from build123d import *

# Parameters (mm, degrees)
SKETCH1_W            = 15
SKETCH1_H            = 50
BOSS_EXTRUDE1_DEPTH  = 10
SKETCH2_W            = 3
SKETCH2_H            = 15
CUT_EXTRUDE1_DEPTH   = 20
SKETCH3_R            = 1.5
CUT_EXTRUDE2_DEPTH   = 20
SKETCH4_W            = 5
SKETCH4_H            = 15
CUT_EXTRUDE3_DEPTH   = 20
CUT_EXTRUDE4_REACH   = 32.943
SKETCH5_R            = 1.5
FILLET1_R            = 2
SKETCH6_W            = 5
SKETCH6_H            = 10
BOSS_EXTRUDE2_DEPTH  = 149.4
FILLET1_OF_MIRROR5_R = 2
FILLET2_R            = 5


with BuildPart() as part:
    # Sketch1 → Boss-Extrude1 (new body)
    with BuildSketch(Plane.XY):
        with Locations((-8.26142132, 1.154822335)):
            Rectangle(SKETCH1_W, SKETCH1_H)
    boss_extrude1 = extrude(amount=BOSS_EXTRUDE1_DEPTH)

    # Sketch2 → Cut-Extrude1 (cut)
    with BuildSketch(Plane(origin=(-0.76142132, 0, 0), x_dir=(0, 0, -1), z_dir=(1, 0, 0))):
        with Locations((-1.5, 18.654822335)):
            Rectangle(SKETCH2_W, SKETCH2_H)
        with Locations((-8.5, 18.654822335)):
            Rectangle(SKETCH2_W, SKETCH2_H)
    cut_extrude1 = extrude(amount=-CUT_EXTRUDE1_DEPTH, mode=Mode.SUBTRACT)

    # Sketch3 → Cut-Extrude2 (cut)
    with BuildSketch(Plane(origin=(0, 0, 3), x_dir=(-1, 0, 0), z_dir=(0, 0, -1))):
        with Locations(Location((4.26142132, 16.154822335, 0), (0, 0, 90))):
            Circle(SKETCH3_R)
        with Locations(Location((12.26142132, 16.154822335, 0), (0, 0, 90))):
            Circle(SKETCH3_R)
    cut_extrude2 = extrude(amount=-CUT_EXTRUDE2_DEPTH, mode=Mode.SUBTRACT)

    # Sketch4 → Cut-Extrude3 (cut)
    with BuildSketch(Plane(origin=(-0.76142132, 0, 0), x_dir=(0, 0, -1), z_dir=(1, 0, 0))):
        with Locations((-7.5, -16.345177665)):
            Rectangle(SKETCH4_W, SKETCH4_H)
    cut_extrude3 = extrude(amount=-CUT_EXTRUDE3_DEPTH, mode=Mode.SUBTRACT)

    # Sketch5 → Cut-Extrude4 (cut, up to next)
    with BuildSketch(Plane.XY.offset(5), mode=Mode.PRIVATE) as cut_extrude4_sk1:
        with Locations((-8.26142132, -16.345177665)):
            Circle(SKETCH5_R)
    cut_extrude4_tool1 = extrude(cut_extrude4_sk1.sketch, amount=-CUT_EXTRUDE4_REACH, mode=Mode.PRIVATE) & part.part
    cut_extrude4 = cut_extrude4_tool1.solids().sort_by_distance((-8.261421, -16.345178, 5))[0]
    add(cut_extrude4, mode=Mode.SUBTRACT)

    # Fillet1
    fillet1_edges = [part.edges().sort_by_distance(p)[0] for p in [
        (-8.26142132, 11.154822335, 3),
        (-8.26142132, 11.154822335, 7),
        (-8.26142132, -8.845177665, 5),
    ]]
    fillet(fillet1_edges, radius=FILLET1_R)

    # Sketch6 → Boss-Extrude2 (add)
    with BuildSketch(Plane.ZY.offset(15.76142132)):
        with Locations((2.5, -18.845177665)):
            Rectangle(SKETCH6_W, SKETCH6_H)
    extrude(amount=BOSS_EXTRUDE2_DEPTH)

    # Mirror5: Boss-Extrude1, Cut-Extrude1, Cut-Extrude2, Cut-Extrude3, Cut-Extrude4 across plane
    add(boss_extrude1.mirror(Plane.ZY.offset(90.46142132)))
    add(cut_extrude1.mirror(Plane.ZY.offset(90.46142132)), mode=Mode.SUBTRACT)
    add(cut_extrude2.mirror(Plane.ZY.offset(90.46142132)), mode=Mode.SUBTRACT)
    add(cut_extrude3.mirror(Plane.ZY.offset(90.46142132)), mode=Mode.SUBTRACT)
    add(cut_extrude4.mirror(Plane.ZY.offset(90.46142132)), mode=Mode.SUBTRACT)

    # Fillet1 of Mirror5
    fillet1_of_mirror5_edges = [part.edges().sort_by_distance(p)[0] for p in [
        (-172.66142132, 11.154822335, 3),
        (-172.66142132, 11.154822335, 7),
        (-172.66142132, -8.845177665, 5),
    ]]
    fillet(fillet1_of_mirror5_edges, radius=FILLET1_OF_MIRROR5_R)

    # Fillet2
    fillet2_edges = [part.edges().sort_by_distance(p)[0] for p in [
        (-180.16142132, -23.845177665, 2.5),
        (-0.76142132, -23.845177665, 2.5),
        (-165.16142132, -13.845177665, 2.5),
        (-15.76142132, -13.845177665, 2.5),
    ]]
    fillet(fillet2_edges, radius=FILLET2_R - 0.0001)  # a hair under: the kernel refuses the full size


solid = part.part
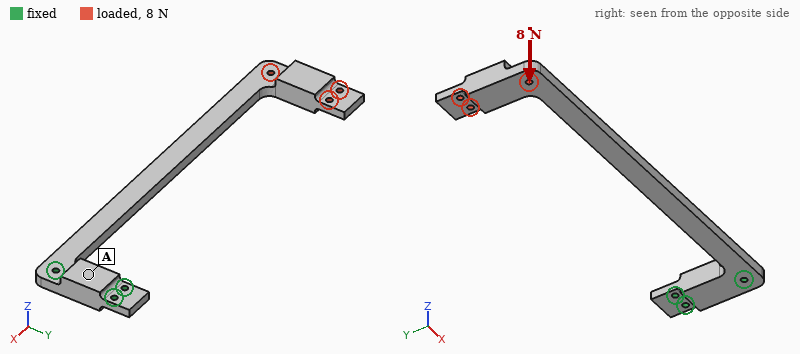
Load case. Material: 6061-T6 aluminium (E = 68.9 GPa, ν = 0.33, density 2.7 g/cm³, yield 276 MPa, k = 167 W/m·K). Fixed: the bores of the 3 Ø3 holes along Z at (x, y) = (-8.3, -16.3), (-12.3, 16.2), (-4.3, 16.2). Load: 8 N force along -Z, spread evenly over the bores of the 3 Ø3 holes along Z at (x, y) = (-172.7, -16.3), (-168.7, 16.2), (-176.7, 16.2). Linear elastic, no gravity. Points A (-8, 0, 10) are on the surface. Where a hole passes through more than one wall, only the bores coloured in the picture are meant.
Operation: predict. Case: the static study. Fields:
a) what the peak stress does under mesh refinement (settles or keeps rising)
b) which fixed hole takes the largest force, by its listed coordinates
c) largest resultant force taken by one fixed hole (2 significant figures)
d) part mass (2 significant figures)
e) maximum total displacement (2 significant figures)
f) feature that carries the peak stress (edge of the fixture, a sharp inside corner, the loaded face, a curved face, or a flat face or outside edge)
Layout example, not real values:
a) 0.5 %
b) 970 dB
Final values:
a) keeps rising
b) (-4.3, 16.2)
c) 30 N
d) 47 g
e) 1.9 mm
f) edge of the fixture
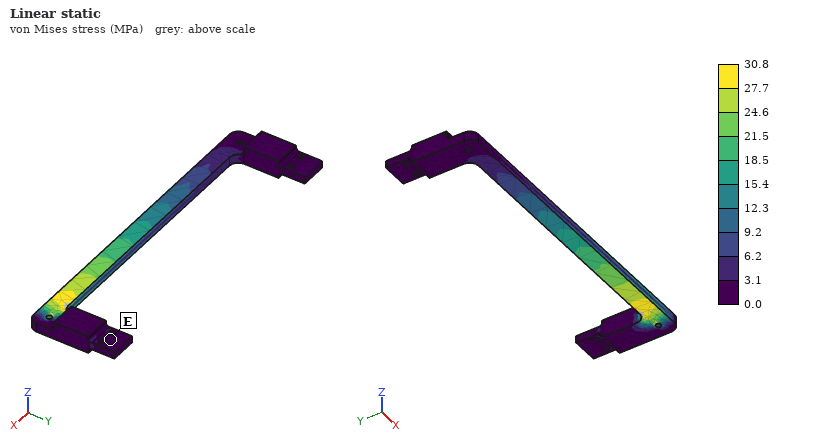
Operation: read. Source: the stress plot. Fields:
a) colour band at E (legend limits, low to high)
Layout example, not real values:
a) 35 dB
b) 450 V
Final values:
a) 0.0 to 3.1 MPa
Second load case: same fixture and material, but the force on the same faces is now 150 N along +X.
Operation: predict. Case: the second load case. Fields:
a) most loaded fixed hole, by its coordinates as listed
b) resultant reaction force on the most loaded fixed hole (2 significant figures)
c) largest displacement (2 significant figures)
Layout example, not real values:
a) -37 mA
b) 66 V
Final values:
a) (-4.3, 16.2)
b) 100 N
c) 1.9 mm
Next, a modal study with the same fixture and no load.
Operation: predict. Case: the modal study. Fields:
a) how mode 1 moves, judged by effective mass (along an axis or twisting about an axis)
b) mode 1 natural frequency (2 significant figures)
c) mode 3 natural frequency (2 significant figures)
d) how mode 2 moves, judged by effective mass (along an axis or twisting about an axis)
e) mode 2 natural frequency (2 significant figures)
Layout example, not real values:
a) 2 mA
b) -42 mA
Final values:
a) along Z
b) 84 Hz
c) 550 Hz
d) along Y
e) 170 Hz
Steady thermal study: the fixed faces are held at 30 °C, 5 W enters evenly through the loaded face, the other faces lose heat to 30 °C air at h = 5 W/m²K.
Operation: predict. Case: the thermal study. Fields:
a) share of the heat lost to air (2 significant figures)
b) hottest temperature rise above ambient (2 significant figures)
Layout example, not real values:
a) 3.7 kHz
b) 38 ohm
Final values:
a) 32 %
b) 75 K
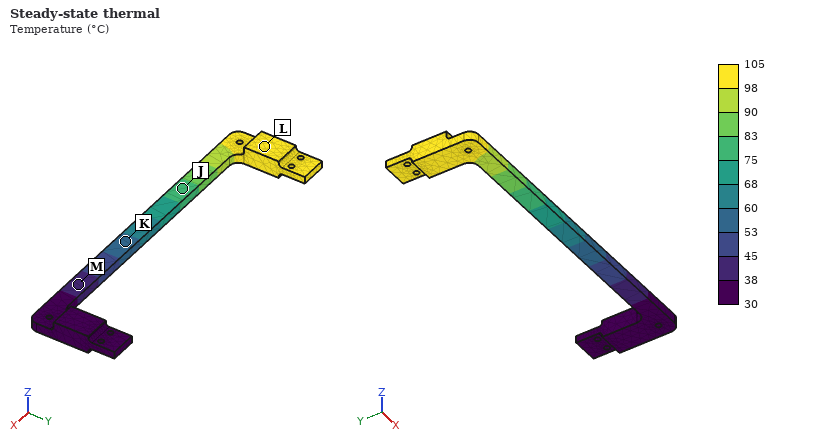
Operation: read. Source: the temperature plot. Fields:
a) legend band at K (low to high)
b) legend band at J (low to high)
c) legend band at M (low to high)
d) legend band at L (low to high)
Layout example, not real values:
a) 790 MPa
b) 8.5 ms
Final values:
a) 53 to 60 °C
b) 75 to 83 °C
c) 38 to 45 °C
d) 98 to 105 °C
